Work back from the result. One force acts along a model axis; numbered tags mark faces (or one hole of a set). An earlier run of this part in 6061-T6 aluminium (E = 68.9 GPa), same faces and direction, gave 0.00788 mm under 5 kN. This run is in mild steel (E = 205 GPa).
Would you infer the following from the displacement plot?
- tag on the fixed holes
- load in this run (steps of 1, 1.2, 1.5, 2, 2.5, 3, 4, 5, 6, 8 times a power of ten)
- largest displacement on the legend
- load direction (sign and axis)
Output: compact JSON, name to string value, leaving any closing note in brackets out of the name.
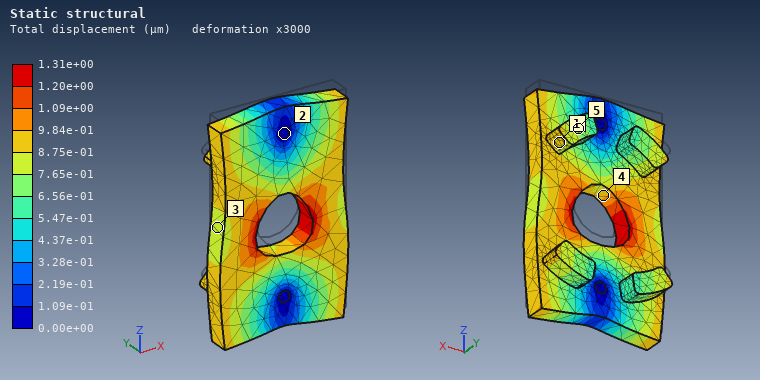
{"tag on the fixed holes": "2", "load in this run": "2.5 kN", "largest displacement on the legend": "1.31e+00 µm", "load direction": "-Z"}
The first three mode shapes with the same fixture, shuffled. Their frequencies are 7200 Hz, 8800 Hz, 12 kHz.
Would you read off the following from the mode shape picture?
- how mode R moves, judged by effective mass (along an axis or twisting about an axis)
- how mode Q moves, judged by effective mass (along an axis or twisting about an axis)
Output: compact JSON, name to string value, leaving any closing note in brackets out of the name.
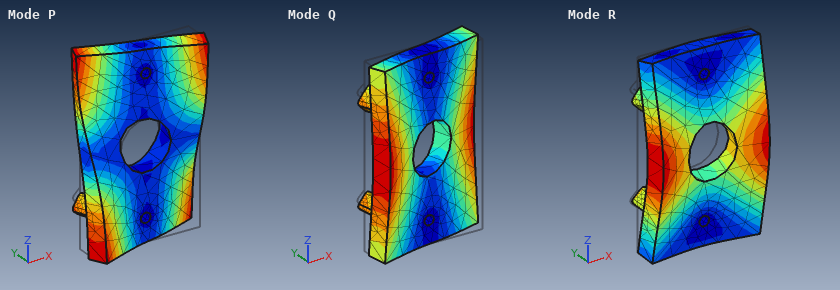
{"how mode R moves, judged by effective mass": "along Y", "how mode Q moves, judged by effective mass": "twisting about Z"}
